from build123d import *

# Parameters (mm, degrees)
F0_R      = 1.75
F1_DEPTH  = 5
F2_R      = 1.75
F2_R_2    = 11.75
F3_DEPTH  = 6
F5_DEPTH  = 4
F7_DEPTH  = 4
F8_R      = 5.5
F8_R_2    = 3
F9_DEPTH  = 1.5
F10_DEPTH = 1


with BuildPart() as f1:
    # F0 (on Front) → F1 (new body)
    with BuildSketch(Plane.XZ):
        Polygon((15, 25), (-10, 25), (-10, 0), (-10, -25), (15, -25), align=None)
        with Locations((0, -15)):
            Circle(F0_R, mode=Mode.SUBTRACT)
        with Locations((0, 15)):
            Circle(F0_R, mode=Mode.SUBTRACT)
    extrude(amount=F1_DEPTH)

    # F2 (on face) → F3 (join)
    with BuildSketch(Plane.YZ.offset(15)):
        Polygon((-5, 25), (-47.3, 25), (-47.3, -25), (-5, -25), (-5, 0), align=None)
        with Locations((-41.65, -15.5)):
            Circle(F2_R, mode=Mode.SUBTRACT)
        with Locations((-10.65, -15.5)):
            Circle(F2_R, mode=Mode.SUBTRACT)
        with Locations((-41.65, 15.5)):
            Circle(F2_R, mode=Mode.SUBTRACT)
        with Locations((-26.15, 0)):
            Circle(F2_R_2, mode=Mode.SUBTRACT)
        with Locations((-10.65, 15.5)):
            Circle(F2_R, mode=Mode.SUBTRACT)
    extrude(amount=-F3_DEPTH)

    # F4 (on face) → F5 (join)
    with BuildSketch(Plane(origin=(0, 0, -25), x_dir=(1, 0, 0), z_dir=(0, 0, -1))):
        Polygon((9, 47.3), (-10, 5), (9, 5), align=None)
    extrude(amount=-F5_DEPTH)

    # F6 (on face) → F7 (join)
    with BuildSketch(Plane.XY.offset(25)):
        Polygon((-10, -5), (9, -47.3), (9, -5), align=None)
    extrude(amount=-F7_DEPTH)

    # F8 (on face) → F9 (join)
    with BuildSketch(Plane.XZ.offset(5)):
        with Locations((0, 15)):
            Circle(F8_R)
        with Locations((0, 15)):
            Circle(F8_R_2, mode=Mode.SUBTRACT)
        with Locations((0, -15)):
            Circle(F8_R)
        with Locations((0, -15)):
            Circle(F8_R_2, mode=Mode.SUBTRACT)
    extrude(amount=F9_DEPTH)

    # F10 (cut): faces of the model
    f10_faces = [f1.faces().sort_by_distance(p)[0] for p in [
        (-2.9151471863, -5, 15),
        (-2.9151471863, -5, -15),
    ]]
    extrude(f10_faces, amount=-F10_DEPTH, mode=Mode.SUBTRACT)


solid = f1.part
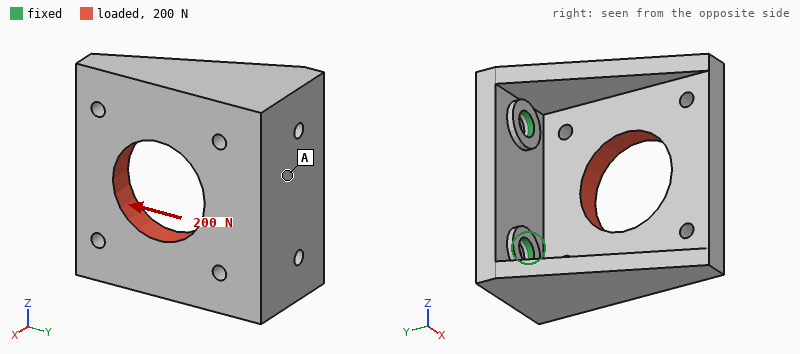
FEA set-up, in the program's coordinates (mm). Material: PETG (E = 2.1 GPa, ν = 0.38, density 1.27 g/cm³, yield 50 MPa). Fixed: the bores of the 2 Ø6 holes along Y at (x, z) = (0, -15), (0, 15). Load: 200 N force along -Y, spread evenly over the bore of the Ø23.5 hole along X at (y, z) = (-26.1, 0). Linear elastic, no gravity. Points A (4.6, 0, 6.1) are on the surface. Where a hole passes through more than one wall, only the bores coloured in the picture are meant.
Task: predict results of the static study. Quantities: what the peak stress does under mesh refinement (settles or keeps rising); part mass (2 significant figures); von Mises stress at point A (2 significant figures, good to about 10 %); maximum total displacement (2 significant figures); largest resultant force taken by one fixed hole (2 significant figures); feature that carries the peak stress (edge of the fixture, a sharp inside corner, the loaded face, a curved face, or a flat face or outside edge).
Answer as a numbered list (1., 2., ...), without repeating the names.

1. keeps rising
2. 25 g
3. 2.9 MPa
4. 0.64 mm
5. 100 N
6. edge of the fixture
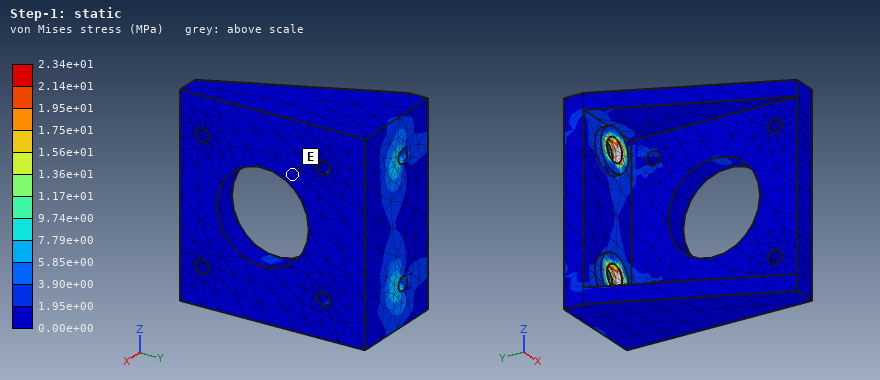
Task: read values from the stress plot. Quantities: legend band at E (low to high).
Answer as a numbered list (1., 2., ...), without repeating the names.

1. 0.00e+00 to 1.95e+00 MPa
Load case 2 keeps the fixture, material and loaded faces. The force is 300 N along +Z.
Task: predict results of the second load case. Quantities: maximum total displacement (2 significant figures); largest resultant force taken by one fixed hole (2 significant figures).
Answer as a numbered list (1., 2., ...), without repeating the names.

1. 0.69 mm
2. 250 N
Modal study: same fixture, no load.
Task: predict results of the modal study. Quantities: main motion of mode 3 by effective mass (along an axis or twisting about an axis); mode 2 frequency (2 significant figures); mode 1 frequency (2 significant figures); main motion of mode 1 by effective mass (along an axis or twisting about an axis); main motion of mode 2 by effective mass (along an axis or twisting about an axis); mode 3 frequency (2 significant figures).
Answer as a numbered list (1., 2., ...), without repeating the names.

1. along Z
2. 910 Hz
3. 570 Hz
4. along X
5. along Z
6. 2000 Hz
